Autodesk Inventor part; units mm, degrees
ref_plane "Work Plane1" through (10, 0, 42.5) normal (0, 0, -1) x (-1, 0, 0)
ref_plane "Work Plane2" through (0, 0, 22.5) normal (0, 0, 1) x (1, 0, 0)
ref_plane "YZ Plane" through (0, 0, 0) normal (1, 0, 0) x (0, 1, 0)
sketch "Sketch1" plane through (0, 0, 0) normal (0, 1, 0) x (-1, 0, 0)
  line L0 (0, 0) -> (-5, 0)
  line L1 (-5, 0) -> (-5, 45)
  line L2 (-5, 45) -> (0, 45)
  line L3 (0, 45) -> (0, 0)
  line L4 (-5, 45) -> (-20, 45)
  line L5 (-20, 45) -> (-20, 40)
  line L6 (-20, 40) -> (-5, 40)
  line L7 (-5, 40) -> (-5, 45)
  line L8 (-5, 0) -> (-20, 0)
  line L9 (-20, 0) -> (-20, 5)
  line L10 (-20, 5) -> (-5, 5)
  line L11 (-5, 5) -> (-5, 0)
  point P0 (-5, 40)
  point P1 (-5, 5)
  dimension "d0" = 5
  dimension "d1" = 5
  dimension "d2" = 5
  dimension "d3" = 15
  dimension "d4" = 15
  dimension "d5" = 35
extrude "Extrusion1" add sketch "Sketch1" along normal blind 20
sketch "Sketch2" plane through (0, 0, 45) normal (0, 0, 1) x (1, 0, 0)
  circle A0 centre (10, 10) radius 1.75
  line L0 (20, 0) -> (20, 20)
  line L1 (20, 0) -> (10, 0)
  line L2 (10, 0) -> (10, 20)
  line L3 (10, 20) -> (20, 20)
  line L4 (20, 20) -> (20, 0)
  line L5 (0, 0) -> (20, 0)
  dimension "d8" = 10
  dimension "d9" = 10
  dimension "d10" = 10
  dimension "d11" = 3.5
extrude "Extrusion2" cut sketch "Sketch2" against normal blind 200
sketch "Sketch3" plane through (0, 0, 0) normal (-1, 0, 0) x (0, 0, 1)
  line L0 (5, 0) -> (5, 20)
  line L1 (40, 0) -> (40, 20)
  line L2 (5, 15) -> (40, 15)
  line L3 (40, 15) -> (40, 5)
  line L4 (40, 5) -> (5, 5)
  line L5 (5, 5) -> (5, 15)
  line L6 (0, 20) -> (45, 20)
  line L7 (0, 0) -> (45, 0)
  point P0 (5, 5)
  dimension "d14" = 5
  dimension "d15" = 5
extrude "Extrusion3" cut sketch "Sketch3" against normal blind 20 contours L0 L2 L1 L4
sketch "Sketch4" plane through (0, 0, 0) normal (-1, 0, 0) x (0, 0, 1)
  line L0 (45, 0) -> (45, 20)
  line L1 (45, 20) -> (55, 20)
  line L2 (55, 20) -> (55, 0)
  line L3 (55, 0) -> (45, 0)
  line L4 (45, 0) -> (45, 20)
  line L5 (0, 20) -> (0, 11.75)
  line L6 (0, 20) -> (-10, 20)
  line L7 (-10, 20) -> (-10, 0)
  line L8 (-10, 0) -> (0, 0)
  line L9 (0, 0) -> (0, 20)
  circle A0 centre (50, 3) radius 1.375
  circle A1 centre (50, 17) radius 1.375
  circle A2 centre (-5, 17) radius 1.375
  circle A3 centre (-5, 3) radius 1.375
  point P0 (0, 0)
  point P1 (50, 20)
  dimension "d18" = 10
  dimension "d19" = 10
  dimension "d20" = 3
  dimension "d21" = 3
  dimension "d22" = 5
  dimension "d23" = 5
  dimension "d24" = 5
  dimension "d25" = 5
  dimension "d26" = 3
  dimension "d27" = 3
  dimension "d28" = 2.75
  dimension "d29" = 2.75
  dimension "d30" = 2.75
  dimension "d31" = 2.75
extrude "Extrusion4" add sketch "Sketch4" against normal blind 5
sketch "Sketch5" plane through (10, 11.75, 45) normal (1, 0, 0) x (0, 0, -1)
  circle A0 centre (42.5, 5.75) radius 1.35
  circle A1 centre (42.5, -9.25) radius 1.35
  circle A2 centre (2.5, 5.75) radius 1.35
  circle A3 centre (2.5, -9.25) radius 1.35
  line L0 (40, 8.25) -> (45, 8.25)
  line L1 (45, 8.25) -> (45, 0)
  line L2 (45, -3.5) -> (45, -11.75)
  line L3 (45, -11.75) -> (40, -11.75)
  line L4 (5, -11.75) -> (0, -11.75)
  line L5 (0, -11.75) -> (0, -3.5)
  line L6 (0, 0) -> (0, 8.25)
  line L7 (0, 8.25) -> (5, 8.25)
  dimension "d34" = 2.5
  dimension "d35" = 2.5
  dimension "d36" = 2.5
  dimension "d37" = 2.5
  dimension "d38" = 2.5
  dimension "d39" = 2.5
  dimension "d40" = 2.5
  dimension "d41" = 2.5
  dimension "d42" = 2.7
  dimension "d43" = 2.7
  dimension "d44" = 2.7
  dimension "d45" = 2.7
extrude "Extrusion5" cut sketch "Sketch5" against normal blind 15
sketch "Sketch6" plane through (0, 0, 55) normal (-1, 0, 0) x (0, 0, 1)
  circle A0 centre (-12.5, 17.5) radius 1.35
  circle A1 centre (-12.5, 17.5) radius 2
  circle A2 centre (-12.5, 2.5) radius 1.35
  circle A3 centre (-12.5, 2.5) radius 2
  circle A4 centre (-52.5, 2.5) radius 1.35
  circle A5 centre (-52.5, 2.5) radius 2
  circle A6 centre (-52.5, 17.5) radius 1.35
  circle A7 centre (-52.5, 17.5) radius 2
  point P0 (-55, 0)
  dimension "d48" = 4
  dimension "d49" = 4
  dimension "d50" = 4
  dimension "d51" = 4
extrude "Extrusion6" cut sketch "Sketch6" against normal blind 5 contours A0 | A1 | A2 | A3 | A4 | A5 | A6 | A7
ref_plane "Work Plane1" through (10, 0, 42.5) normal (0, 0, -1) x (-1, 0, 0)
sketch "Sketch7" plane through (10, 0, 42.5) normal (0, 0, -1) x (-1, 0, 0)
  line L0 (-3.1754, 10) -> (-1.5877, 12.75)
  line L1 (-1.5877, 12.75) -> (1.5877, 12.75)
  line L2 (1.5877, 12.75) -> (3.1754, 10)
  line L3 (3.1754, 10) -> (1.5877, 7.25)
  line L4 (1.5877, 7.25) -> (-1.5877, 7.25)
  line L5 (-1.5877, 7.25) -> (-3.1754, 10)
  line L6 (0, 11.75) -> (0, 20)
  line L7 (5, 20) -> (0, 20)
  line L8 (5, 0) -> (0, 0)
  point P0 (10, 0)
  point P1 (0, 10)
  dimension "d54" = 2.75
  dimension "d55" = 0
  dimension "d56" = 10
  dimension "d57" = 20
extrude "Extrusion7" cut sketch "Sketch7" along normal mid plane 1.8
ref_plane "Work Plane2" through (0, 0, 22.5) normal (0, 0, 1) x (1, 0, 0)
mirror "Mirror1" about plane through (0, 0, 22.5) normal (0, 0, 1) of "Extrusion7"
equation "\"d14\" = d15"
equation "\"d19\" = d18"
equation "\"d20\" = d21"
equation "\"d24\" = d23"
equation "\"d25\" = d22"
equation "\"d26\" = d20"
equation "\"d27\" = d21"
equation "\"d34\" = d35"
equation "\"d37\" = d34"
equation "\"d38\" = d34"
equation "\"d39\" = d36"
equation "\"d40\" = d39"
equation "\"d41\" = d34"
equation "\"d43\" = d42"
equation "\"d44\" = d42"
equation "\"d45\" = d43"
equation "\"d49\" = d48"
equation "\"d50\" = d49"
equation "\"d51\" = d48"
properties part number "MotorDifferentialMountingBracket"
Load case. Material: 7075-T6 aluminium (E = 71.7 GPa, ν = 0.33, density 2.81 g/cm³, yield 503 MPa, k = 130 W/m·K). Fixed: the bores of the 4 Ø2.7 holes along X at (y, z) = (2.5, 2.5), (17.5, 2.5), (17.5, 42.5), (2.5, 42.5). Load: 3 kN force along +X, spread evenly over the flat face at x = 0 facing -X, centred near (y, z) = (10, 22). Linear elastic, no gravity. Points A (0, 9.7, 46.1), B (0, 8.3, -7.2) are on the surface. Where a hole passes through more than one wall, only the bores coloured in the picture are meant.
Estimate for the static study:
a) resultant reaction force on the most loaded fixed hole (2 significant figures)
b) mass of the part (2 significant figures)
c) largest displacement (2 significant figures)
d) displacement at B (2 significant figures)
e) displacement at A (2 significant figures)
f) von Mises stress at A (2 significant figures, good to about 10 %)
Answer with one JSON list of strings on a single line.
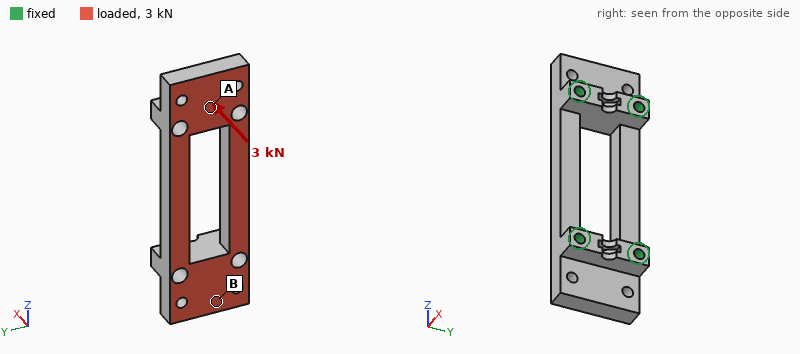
["780 N", "15 g", "35 µm", "17 µm", "7.9 µm", "30 MPa"]
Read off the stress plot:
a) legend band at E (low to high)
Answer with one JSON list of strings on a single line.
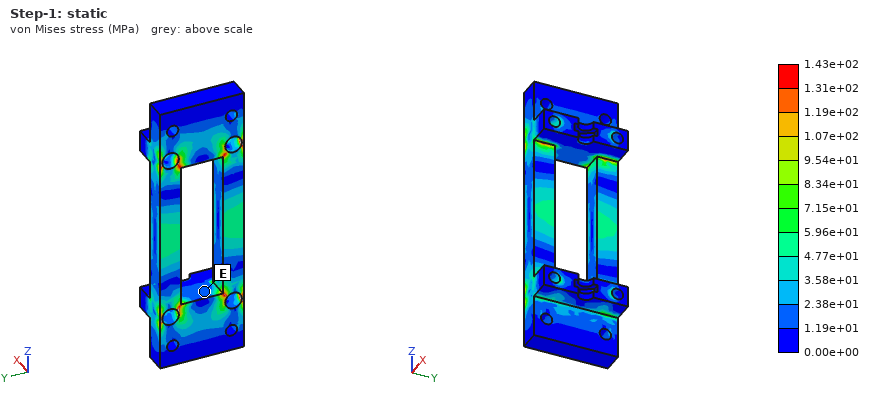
["1.19e+01 to 2.38e+01 MPa"]
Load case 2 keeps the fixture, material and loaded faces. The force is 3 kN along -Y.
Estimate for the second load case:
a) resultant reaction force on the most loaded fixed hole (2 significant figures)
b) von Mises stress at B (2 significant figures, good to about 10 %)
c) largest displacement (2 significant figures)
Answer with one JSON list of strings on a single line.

["980 N", "12 MPa", "49 µm"]
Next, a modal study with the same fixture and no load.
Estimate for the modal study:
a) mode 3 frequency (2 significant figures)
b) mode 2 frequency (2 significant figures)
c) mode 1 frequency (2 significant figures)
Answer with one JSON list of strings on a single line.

["14 kHz", "14 kHz", "13 kHz"]
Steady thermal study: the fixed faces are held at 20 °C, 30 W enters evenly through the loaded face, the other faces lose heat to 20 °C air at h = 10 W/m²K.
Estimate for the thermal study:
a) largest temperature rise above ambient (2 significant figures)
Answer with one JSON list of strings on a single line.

["16 K"]
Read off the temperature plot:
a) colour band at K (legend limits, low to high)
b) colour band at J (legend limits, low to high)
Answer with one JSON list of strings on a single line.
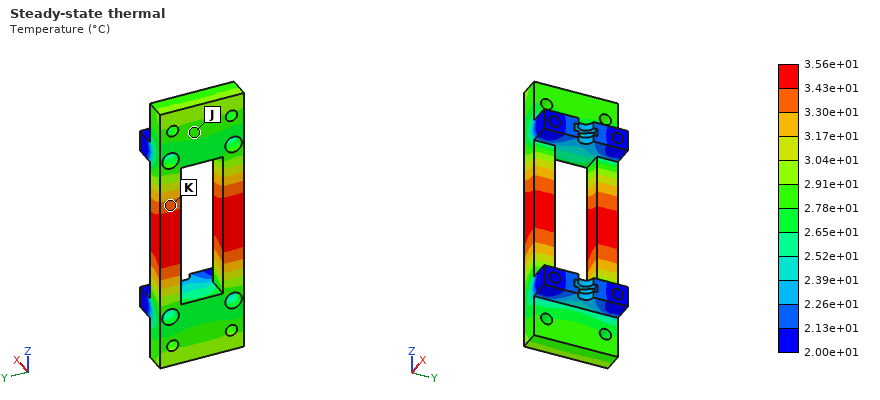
["3.30e+01 to 3.43e+01 °C", "2.78e+01 to 2.91e+01 °C"]
